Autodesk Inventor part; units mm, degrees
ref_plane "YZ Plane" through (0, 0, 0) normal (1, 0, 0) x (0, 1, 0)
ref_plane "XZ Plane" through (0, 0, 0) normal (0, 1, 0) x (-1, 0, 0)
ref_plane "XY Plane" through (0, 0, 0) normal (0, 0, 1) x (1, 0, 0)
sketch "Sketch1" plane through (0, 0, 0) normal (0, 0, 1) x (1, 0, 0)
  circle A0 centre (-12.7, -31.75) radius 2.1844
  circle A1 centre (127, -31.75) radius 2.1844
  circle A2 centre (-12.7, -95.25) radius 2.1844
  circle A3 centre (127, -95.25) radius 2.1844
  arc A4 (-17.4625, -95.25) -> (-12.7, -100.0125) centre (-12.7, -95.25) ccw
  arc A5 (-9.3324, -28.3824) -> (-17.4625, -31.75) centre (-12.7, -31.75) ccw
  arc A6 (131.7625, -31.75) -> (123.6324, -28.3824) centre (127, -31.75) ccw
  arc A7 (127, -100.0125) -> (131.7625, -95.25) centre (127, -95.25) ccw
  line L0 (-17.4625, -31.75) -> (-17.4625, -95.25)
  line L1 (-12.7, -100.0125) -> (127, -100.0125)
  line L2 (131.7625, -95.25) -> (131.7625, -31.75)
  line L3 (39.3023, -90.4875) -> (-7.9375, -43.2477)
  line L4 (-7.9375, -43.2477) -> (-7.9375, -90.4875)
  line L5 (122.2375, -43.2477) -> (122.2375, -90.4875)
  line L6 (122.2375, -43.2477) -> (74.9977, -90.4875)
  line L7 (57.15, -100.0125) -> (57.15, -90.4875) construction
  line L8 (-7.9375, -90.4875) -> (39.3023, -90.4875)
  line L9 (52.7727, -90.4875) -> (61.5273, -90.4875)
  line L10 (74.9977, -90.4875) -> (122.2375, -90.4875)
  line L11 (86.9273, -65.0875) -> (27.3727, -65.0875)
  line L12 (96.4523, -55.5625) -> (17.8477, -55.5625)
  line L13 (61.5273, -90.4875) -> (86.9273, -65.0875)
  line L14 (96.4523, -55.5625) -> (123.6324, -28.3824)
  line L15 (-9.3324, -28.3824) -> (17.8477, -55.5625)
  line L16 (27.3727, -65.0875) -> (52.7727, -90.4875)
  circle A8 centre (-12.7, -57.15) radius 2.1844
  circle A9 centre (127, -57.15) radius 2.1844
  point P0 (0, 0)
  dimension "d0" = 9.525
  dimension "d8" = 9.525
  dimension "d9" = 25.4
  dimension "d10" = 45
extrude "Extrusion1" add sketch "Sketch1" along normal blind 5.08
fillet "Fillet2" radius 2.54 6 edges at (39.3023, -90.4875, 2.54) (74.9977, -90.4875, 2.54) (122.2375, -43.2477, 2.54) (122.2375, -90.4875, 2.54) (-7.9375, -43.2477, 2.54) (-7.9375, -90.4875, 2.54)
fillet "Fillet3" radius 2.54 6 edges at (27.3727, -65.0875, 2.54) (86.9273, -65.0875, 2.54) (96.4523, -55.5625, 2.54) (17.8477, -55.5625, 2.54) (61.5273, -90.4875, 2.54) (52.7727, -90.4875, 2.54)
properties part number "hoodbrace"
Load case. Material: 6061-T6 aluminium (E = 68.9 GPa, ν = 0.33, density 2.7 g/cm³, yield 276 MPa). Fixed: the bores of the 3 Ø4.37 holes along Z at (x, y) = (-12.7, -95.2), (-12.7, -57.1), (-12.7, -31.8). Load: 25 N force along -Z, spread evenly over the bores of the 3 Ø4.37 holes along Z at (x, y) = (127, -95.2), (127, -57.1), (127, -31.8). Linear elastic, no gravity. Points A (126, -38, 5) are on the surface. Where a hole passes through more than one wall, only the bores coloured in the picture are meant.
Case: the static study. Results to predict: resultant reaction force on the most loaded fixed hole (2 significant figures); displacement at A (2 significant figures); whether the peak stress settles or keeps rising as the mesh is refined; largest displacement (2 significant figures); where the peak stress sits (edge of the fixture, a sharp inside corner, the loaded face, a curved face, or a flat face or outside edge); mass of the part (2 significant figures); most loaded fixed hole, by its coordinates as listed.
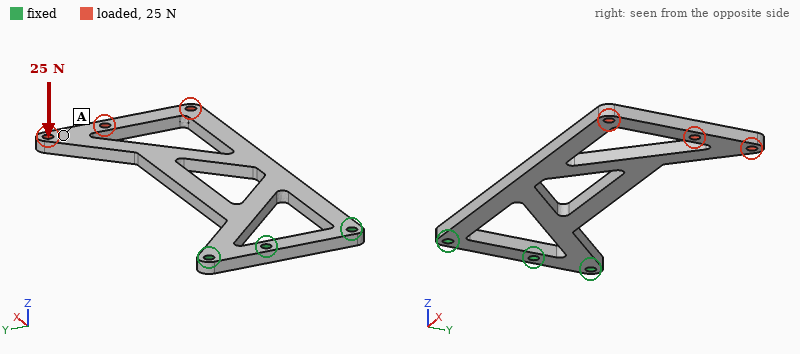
23 N
1.6 mm
keeps rising
1.7 mm
edge of the fixture
64 g
(-12.7, -31.8)
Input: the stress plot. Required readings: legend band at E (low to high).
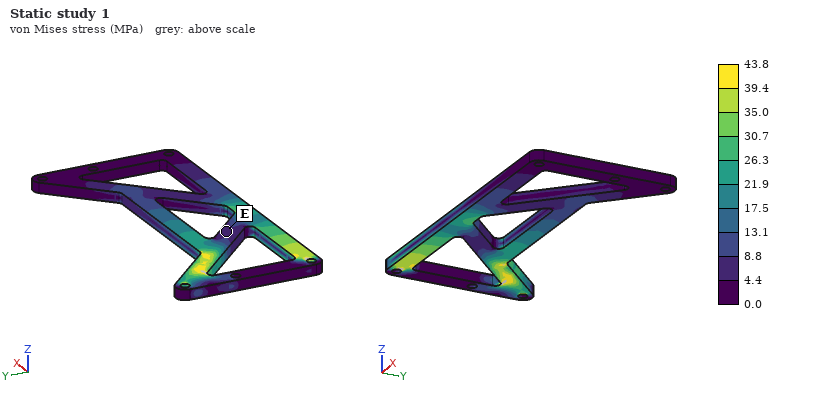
4.4 to 8.8 MPa
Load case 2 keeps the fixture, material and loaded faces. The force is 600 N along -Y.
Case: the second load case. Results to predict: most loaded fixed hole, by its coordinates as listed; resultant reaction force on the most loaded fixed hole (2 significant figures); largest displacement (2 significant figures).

(-12.7, -95.2)
1.6 kN
0.65 mm
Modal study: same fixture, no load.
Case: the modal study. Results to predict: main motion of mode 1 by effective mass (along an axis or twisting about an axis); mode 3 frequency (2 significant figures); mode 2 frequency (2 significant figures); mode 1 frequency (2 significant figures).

along Z
1000 Hz
650 Hz
150 Hz
